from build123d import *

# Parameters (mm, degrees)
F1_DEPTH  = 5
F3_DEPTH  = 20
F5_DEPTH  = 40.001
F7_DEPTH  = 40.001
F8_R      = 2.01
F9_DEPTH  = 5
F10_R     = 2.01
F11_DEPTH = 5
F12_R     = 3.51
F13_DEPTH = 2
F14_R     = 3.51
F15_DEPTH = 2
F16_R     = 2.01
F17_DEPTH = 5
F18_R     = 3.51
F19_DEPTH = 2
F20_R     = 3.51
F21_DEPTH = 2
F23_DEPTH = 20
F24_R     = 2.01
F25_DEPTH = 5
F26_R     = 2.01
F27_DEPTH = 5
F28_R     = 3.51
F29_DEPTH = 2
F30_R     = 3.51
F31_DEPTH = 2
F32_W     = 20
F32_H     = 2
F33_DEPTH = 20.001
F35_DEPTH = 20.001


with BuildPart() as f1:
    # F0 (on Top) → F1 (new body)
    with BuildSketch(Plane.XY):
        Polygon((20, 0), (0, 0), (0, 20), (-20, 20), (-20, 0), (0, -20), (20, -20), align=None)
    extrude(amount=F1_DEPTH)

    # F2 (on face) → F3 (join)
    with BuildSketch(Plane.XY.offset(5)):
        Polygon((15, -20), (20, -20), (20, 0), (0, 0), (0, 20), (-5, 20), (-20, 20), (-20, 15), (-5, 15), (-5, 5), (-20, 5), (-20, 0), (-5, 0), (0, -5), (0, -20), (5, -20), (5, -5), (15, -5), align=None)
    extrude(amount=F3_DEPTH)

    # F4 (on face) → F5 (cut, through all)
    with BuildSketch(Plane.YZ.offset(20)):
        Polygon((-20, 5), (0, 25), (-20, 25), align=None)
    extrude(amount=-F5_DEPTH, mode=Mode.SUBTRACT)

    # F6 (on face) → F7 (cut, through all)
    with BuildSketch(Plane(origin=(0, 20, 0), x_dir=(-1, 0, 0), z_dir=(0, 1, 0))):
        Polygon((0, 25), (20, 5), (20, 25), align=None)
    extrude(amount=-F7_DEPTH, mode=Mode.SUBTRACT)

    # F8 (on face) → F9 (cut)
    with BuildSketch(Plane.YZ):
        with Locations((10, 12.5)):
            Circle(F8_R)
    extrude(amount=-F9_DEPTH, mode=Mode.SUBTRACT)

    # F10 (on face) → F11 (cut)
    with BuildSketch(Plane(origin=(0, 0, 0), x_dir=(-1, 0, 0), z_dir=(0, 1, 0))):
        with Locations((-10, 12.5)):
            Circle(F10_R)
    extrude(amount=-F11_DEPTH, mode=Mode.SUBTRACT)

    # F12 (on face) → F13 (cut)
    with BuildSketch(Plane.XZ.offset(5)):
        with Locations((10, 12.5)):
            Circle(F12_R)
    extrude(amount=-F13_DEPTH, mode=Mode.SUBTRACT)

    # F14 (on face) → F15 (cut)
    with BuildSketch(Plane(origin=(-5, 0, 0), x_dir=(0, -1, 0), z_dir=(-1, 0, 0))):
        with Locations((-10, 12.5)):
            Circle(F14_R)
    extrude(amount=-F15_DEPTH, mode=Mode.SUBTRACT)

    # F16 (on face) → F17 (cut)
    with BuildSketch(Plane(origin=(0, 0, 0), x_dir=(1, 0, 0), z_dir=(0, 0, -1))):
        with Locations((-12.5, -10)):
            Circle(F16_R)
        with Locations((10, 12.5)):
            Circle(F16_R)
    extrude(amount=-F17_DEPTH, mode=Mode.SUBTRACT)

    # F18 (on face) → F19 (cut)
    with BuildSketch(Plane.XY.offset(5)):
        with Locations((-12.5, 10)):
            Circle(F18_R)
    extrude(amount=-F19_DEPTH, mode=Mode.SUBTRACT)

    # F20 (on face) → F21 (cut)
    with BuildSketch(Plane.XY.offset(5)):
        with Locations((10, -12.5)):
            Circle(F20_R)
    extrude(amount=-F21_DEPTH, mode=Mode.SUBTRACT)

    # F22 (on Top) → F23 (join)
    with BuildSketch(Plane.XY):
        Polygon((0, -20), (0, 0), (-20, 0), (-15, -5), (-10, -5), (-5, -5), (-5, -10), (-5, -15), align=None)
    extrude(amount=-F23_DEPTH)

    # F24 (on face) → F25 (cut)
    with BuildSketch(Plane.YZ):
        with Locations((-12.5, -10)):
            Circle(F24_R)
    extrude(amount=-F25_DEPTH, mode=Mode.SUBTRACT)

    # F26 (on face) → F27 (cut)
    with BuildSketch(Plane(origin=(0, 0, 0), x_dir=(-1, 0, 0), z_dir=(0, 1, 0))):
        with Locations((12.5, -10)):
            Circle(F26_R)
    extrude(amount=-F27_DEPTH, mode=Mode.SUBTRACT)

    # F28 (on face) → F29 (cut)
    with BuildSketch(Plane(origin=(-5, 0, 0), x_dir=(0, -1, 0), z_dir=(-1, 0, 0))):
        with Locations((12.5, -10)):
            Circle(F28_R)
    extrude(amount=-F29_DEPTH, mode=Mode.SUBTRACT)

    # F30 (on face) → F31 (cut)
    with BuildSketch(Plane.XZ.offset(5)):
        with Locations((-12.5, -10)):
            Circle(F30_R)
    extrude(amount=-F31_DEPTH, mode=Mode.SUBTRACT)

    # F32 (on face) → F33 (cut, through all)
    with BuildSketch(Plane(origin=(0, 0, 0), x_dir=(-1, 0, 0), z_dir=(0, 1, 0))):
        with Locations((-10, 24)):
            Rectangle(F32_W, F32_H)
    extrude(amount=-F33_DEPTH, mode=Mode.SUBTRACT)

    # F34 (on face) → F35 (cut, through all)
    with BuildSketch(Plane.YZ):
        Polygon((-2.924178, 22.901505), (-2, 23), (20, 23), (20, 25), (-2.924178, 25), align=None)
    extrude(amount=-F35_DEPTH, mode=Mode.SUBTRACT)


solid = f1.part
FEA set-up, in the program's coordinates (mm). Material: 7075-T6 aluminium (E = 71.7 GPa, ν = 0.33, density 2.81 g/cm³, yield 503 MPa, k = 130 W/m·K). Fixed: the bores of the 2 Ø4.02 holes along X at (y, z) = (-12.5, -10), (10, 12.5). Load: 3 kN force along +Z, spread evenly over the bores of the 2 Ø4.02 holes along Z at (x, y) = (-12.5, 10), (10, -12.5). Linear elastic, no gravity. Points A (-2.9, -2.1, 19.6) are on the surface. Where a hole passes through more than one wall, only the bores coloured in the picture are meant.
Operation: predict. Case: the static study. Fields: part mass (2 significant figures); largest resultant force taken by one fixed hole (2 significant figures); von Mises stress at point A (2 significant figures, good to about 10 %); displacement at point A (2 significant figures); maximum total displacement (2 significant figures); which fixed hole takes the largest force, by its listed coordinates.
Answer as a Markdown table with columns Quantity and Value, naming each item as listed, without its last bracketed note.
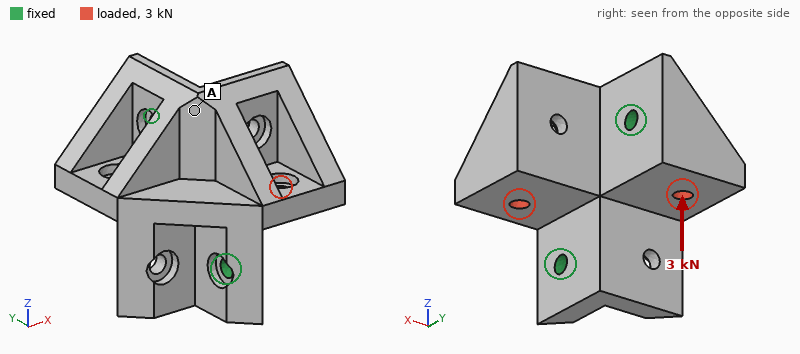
| Quantity | Value |
|---|---|
| part mass | 37 g |
| largest resultant force taken by one fixed hole | 1.6 kN |
| von Mises stress at point A | 22 MPa |
| displacement at point A | 19 µm |
| maximum total displacement | 62 µm |
| which fixed hole takes the largest force, by its listed coordinates | (-12.5, -10) |
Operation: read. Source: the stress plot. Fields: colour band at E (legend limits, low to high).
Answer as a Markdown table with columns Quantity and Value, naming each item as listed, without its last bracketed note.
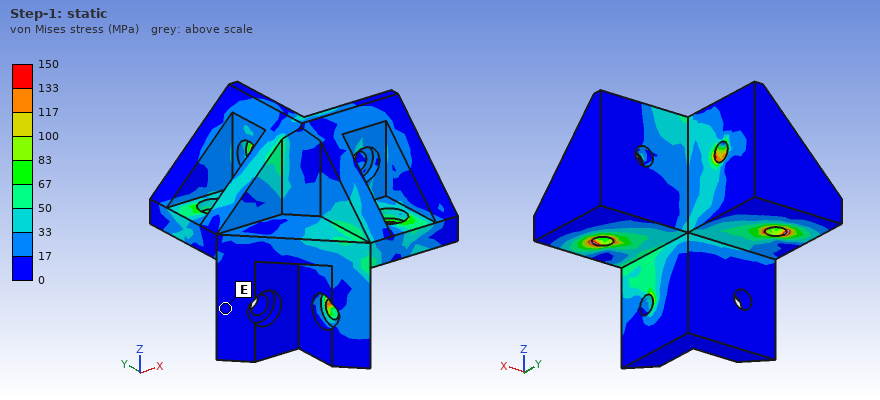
| Quantity | Value |
|---|---|
| colour band at E | 0 to 17 MPa |
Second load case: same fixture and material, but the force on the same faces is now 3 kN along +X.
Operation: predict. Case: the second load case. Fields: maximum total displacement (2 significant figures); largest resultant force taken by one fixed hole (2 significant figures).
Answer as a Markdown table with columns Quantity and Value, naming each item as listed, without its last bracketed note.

| Quantity | Value |
|---|---|
| maximum total displacement | 54 µm |
| largest resultant force taken by one fixed hole | 1.7 kN |
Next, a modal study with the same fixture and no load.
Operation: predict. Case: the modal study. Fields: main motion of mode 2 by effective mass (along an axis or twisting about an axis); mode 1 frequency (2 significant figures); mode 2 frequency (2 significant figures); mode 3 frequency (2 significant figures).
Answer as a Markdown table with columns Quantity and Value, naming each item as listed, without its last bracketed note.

| Quantity | Value |
|---|---|
| main motion of mode 2 by effective mass | along Y |
| mode 1 frequency | 3800 Hz |
| mode 2 frequency | 9200 Hz |
| mode 3 frequency | 10 kHz |
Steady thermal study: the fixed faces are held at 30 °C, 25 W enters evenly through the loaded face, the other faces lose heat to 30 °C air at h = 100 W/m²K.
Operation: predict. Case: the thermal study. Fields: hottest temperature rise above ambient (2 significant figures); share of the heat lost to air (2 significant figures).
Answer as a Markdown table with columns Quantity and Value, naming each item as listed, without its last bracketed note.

| Quantity | Value |
|---|---|
| hottest temperature rise above ambient | 20 K |
| share of the heat lost to air | 22 % |
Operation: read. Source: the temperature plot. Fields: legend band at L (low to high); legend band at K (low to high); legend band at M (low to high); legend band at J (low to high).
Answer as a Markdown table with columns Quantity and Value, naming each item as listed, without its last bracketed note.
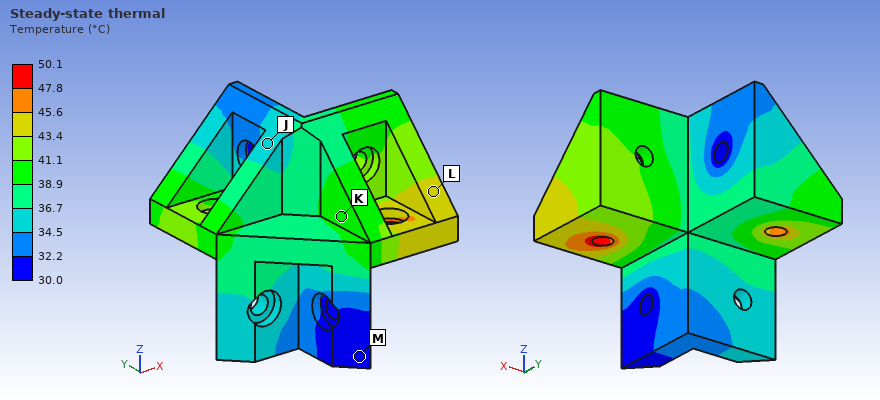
| Quantity | Value |
|---|---|
| legend band at L | 43.4 to 45.6 °C |
| legend band at K | 38.9 to 41.1 °C |
| legend band at M | 30.0 to 32.2 °C |
| legend band at J | 34.5 to 36.7 °C |
